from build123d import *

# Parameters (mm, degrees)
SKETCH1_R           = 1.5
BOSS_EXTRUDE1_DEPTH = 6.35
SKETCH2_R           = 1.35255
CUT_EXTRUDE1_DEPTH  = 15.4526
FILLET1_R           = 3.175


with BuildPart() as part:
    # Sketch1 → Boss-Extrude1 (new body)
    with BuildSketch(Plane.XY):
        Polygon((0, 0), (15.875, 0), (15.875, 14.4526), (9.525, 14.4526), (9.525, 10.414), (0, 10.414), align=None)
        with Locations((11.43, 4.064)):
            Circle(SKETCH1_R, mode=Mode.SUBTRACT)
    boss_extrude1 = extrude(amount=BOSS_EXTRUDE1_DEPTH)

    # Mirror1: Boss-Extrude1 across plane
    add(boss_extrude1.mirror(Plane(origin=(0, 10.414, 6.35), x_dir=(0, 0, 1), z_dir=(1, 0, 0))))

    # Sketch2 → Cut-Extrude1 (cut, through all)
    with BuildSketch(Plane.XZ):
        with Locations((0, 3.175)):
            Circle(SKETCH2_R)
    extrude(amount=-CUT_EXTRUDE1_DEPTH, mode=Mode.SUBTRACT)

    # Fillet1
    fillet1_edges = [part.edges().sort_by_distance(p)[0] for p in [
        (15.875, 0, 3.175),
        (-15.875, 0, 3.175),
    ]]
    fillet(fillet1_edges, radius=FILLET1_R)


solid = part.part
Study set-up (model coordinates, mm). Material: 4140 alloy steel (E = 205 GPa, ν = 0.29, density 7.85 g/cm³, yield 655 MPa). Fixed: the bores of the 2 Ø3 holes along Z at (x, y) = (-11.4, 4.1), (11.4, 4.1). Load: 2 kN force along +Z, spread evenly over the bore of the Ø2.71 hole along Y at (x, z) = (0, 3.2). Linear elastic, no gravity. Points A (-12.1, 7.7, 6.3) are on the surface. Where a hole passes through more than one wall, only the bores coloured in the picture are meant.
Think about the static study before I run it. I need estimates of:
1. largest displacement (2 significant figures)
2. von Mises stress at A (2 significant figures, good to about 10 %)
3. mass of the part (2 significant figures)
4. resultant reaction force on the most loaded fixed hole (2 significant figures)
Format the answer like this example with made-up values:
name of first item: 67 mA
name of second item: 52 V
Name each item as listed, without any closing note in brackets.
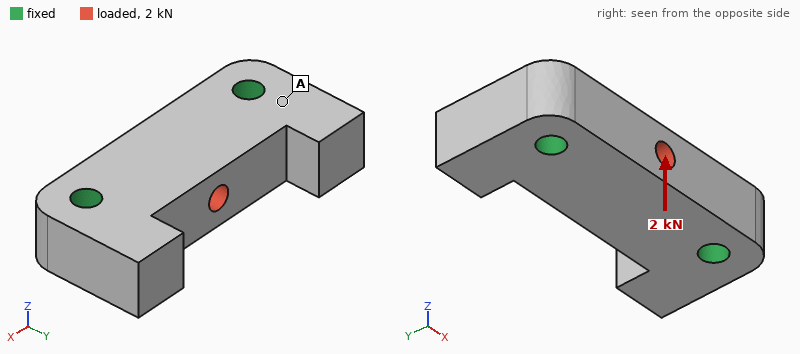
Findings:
largest displacement: 5.9 µm
von Mises stress at A: 27 MPa
mass of the part: 18 g
resultant reaction force on the most loaded fixed hole: 1.0 kN
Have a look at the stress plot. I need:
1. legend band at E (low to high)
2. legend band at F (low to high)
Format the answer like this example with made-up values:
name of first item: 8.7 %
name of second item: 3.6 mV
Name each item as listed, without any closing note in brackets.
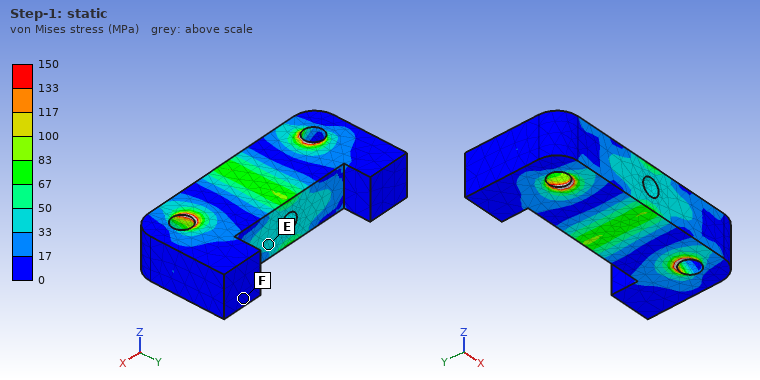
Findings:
legend band at E: 33 to 50 MPa
legend band at F: 0 to 17 MPa
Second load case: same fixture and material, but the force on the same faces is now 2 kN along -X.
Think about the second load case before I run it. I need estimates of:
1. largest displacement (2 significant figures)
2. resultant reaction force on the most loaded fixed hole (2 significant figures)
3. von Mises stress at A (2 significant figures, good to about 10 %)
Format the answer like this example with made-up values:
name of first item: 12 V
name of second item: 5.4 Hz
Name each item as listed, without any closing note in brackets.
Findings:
largest displacement: 1.0 µm
resultant reaction force on the most loaded fixed hole: 1.0 kN
von Mises stress at A: 7.5 MPa
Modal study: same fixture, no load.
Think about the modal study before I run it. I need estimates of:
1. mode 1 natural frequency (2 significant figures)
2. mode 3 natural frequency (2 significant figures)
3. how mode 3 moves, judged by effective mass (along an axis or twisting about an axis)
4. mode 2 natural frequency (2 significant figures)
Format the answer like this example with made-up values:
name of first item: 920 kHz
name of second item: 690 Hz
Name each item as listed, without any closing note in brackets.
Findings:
mode 1 natural frequency: 42 kHz
mode 3 natural frequency: 47 kHz
how mode 3 moves, judged by effective mass: twisting about Y
mode 2 natural frequency: 42 kHz
